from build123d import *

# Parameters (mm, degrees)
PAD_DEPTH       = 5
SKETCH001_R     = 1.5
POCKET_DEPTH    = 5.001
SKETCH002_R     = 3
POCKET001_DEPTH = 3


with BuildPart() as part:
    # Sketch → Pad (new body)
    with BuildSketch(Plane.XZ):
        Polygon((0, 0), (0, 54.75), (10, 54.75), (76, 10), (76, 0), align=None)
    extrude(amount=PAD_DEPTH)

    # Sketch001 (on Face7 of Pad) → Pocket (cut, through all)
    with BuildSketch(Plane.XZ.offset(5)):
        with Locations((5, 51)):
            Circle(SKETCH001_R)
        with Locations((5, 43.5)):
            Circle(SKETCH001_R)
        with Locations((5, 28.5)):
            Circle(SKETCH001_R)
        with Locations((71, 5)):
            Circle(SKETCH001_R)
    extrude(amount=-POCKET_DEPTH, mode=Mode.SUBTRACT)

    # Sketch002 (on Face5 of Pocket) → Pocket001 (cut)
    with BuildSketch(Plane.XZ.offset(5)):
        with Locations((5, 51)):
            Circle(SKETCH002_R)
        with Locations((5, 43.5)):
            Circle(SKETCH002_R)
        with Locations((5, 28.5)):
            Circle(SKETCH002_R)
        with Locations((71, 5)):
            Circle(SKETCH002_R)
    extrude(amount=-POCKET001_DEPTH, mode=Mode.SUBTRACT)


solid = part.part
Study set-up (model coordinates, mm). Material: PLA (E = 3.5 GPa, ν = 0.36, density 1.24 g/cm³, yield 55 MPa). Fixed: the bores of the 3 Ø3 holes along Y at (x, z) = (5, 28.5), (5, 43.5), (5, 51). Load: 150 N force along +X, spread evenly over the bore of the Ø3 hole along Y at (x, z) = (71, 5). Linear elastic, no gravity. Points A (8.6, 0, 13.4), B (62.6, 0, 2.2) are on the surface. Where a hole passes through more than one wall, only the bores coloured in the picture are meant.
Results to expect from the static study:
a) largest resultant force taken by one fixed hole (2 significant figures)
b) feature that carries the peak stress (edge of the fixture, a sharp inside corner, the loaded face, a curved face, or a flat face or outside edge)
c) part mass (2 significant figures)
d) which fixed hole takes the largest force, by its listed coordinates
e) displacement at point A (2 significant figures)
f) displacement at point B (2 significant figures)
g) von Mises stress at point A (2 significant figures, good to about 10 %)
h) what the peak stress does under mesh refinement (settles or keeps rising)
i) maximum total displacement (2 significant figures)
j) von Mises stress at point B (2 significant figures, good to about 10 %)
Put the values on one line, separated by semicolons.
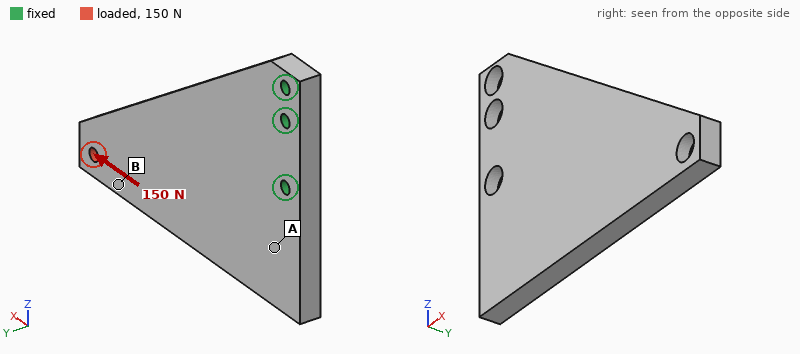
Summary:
300 N; edge of the fixture; 16 g; (5, 28.5); 0.093 mm; 0.31 mm; 2.4 MPa; keeps rising; 0.46 mm; 6.7 MPa
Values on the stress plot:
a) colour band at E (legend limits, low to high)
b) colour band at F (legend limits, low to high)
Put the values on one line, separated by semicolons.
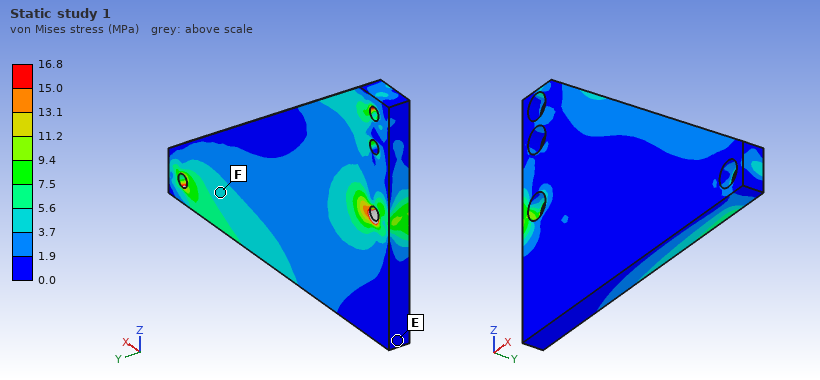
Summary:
0.0 to 1.9 MPa; 3.7 to 5.6 MPa
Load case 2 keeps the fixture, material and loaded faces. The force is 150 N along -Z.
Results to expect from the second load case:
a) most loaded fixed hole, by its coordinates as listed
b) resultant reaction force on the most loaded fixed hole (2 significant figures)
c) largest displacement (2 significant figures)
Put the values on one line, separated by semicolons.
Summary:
(5, 28.5); 460 N; 1.0 mm
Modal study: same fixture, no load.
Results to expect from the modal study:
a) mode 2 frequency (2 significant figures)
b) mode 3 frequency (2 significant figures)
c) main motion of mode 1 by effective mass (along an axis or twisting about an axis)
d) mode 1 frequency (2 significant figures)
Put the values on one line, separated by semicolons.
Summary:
1000 Hz; 1300 Hz; along Y; 250 Hz
